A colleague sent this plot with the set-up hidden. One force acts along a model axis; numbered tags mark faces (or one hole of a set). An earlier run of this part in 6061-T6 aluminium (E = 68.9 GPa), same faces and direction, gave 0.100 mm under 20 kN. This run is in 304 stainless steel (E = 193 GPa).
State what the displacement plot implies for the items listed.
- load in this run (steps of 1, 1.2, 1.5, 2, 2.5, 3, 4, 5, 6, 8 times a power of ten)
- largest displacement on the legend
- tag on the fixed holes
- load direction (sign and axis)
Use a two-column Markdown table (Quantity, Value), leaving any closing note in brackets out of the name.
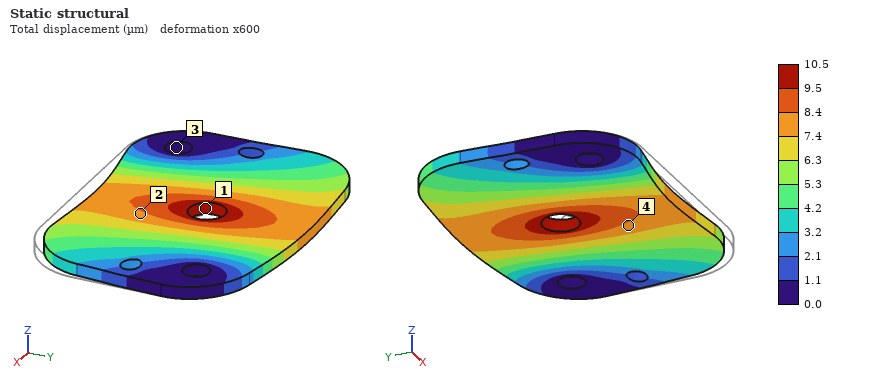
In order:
| Quantity | Value |
|---|---|
| load in this run | 6 kN |
| largest displacement on the legend | 10.5 µm |
| tag on the fixed holes | 3 |
| load direction | +Y |
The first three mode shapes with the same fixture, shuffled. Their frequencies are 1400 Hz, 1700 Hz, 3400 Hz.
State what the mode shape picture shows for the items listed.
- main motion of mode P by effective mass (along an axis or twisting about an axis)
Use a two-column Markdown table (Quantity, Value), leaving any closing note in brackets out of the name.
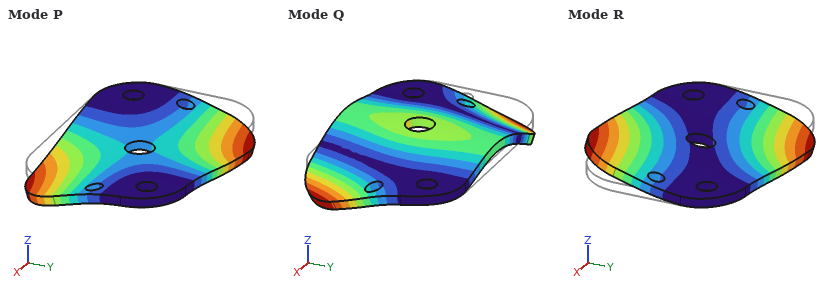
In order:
| Quantity | Value |
|---|---|
| main motion of mode P by effective mass | along Z |
